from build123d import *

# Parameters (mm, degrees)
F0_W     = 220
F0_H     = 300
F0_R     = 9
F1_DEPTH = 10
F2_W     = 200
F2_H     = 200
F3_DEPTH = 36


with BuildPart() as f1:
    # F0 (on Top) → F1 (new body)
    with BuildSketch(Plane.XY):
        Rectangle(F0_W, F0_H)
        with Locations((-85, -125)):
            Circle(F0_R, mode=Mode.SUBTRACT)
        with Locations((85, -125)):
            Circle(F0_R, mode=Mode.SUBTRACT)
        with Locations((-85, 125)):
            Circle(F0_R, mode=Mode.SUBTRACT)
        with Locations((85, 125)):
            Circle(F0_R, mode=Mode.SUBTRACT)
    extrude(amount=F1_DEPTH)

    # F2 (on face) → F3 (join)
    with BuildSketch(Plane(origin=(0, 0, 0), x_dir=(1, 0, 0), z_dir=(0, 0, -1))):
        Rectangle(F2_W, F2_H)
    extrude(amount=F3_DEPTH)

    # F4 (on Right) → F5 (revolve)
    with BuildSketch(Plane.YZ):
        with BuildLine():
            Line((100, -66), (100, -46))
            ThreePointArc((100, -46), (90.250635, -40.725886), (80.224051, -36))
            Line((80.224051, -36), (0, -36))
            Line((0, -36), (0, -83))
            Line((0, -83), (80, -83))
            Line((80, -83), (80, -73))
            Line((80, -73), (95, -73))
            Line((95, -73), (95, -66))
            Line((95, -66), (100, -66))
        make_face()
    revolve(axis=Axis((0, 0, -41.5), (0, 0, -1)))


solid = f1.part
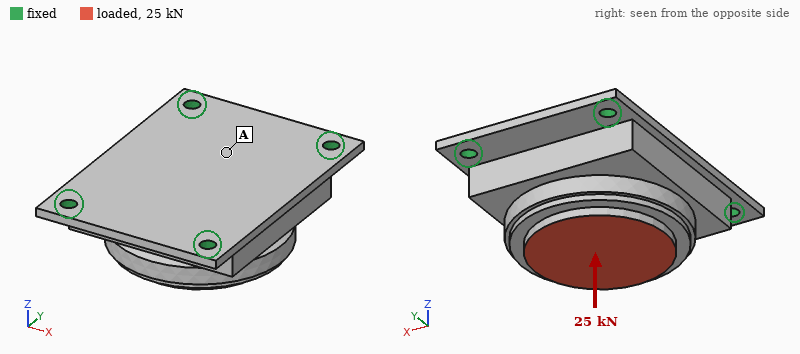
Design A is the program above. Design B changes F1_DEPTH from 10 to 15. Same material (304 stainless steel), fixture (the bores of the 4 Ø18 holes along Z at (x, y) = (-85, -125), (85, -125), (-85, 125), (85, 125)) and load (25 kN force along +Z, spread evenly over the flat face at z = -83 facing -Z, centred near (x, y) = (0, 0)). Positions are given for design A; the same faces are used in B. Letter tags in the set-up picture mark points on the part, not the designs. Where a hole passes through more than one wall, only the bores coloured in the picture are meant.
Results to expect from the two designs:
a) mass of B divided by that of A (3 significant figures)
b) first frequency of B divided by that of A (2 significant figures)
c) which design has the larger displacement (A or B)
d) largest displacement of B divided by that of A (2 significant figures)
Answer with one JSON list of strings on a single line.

["1.10", "1.3", "A", "0.58"]
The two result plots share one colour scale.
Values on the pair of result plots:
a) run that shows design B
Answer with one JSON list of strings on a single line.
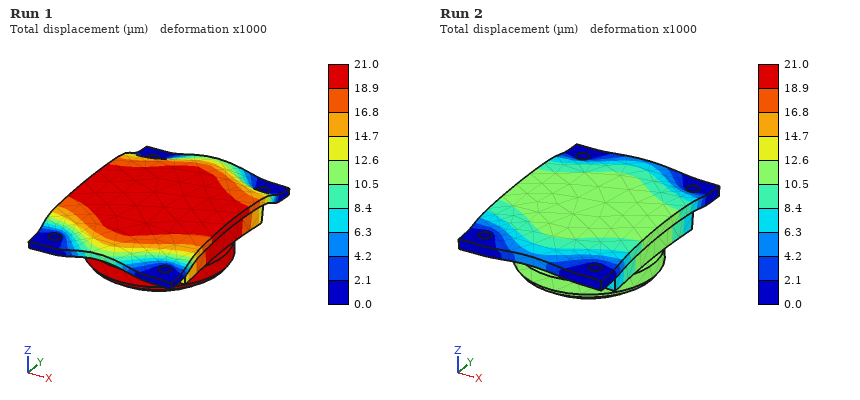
["Run 2"]
